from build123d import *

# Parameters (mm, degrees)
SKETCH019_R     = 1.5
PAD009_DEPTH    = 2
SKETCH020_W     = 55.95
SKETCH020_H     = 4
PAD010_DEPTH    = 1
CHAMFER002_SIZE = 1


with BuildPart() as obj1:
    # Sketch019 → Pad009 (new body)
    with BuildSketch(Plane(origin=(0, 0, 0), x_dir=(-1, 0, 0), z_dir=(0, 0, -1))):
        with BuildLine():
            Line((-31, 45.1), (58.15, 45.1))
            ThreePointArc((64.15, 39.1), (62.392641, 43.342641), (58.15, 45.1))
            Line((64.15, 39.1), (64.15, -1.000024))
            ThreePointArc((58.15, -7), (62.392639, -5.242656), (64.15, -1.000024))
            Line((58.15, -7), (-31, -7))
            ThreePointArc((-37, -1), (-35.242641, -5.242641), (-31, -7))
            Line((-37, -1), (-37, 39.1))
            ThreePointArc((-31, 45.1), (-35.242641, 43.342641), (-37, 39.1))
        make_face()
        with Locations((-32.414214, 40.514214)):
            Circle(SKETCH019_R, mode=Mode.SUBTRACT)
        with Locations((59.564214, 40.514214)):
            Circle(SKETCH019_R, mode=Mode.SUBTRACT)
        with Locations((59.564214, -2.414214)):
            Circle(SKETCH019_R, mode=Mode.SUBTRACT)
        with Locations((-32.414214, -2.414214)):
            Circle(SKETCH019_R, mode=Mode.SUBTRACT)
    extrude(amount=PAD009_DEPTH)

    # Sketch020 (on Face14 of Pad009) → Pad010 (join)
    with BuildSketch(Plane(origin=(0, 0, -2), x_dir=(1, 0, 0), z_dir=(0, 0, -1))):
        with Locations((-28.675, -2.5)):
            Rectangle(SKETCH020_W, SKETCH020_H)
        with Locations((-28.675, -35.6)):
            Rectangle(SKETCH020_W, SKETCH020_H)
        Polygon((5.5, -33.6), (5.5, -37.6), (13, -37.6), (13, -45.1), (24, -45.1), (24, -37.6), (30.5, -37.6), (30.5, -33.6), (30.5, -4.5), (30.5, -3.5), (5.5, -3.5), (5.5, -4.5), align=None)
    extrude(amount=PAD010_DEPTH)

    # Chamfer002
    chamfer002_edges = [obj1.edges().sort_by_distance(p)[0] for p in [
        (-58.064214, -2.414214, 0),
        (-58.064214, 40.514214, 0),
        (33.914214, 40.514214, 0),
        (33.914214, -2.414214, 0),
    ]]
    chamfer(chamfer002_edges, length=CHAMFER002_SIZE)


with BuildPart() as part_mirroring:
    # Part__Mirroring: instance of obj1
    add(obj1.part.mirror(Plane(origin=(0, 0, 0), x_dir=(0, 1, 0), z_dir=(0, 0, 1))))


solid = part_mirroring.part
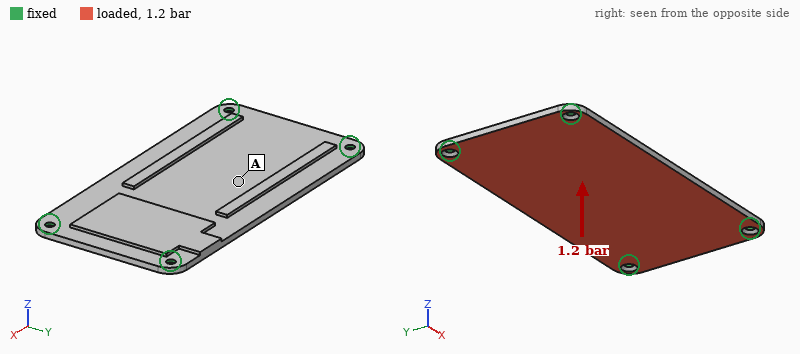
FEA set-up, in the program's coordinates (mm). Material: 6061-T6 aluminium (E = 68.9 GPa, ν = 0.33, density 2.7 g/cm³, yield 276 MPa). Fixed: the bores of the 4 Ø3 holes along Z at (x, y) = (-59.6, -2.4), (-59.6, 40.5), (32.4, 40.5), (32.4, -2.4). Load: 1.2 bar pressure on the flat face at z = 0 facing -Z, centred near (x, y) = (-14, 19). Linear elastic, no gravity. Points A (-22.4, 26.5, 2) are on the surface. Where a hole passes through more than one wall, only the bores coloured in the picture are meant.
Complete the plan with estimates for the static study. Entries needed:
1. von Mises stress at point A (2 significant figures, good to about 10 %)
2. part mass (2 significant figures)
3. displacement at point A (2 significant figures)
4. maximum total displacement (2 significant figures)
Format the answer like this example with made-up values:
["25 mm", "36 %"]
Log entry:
["43 MPa", "32 g", "0.55 mm", "0.60 mm"]
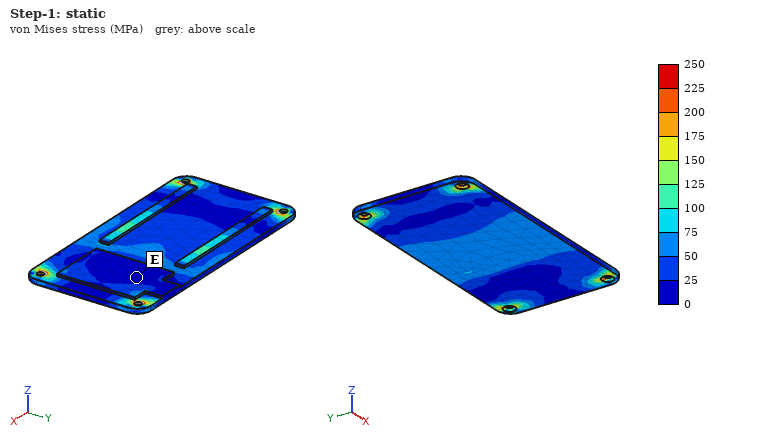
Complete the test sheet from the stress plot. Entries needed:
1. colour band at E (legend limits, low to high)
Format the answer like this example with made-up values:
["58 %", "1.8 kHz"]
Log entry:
["0 to 25 MPa"]
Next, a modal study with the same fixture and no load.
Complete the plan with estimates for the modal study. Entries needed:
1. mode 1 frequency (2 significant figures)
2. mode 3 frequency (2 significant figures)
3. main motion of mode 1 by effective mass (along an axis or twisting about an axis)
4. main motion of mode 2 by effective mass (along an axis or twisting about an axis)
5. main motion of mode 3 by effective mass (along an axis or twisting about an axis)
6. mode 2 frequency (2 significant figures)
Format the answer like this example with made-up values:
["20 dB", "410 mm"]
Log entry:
["1100 Hz", "3000 Hz", "along Z", "twisting about X", "twisting about Y", "2100 Hz"]
